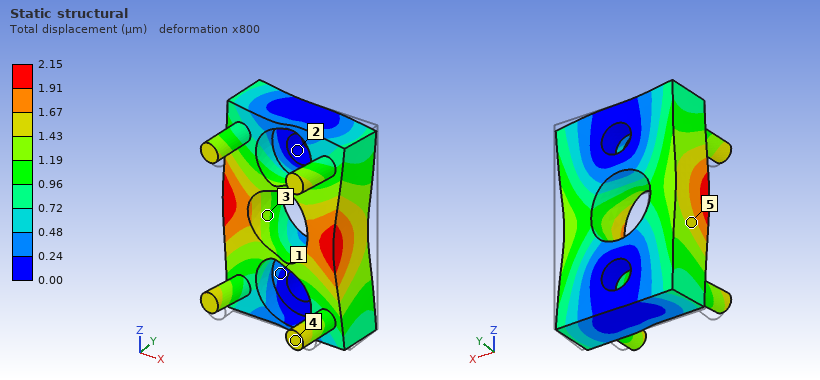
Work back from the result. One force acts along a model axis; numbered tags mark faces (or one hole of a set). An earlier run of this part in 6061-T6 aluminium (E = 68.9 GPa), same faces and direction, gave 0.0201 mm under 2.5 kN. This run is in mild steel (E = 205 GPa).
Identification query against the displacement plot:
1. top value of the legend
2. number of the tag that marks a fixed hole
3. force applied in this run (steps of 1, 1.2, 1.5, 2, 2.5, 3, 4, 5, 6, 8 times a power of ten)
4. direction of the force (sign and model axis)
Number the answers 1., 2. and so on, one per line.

1. 2.15 µm
2. 2
3. 800 N
4. -X
